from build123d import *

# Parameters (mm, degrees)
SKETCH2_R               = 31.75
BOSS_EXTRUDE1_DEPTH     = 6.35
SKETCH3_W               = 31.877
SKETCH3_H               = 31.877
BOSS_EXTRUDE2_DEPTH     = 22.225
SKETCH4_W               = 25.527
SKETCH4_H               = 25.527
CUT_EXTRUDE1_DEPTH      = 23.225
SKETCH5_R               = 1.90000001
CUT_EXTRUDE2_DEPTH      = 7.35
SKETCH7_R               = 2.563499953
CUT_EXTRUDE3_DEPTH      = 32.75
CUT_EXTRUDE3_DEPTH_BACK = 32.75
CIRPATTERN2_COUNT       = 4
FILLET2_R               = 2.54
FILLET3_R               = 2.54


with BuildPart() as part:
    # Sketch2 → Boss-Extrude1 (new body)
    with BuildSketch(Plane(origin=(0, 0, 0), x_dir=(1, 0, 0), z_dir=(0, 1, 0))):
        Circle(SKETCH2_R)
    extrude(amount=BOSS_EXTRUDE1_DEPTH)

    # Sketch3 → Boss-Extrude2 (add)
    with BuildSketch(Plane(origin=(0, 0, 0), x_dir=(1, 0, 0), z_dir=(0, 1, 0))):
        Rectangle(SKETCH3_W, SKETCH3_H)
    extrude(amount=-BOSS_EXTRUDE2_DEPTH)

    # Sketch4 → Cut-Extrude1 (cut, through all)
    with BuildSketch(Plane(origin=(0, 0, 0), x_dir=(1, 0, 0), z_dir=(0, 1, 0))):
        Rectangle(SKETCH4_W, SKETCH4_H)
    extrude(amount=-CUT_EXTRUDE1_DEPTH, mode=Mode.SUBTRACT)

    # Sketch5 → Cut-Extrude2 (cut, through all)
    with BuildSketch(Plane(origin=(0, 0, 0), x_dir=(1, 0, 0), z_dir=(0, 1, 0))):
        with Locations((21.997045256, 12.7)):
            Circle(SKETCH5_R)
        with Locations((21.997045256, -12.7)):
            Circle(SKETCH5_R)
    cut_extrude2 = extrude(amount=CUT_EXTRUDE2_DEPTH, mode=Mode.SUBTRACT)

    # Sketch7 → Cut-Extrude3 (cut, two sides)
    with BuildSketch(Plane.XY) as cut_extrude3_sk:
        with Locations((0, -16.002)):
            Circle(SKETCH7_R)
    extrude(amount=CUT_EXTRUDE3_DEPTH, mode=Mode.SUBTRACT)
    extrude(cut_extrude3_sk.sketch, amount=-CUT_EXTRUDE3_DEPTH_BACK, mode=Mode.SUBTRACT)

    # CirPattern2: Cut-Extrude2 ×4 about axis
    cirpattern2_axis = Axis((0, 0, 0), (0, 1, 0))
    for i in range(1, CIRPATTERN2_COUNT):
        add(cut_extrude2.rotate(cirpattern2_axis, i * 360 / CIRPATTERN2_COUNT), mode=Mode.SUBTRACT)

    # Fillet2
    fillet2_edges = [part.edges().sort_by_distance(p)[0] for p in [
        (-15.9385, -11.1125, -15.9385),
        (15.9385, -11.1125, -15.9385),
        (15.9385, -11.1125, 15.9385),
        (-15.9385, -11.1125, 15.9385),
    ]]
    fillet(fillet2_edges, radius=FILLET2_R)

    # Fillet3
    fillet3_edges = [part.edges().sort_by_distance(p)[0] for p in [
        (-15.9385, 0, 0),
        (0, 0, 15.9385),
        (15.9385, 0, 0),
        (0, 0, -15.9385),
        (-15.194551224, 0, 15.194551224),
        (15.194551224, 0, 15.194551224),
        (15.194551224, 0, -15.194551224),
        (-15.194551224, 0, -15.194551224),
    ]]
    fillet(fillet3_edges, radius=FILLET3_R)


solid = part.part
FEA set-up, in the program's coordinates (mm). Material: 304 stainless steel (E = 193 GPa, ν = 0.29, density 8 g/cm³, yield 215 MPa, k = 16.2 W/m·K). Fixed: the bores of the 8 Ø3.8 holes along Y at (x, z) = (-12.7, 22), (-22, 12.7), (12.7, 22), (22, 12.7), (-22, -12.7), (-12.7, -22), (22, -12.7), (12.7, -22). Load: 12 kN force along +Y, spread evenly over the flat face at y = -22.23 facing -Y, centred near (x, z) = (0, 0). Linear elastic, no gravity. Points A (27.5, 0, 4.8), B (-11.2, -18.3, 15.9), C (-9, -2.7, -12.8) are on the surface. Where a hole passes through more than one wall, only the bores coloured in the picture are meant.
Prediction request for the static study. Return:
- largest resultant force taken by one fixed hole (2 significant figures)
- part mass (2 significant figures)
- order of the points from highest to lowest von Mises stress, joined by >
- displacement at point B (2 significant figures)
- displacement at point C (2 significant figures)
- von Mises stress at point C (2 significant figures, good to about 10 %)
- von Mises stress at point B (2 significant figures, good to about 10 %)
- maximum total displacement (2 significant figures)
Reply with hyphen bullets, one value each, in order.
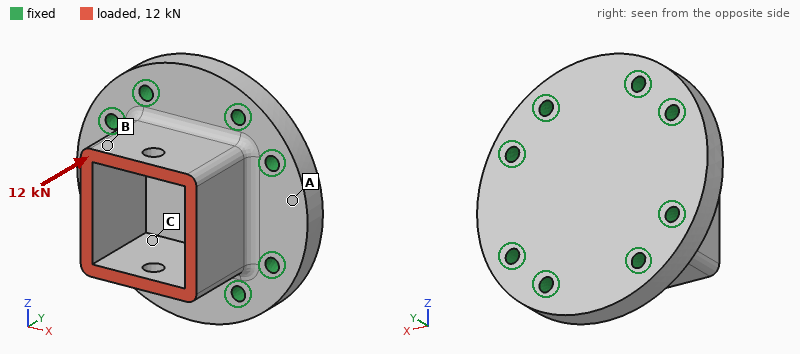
- 1.6 kN
- 220 g
- B > C > A
- 7.1 µm
- 4.5 µm
- 23 MPa
- 33 MPa
- 8.9 µm
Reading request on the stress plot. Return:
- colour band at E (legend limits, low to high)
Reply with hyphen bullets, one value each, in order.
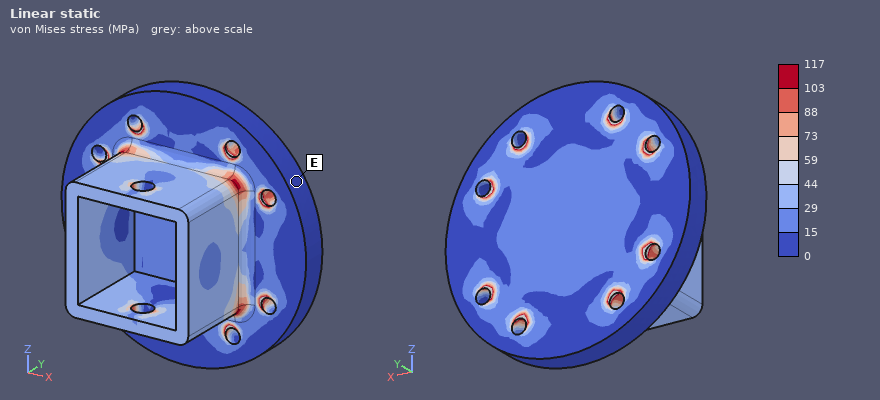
- 0 to 15 MPa
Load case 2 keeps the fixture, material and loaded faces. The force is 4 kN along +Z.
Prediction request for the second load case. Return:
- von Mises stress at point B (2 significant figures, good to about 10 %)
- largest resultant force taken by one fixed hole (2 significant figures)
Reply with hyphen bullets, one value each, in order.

- 83 MPa
- 1.2 kN
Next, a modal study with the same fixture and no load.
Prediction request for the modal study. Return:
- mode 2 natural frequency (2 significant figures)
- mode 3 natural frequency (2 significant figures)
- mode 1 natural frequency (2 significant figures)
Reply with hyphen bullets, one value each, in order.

- 15 kHz
- 15 kHz
- 13 kHz
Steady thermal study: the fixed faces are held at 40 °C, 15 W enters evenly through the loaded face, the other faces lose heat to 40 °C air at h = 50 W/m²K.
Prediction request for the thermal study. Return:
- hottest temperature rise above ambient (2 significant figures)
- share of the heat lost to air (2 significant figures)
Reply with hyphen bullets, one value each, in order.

- 52 K
- 48 %
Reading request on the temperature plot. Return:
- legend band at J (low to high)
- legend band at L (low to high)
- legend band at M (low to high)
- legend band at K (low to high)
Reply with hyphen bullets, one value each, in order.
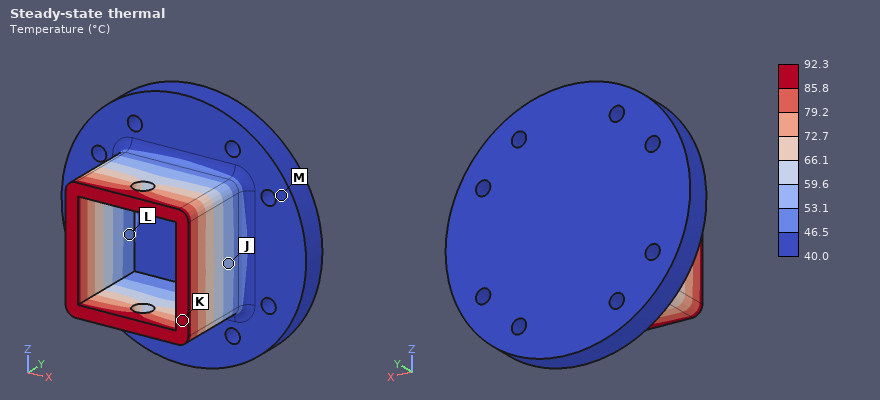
- 53.1 to 59.6 °C
- 46.5 to 53.1 °C
- 40.0 to 46.5 °C
- 85.8 to 92.3 °C
